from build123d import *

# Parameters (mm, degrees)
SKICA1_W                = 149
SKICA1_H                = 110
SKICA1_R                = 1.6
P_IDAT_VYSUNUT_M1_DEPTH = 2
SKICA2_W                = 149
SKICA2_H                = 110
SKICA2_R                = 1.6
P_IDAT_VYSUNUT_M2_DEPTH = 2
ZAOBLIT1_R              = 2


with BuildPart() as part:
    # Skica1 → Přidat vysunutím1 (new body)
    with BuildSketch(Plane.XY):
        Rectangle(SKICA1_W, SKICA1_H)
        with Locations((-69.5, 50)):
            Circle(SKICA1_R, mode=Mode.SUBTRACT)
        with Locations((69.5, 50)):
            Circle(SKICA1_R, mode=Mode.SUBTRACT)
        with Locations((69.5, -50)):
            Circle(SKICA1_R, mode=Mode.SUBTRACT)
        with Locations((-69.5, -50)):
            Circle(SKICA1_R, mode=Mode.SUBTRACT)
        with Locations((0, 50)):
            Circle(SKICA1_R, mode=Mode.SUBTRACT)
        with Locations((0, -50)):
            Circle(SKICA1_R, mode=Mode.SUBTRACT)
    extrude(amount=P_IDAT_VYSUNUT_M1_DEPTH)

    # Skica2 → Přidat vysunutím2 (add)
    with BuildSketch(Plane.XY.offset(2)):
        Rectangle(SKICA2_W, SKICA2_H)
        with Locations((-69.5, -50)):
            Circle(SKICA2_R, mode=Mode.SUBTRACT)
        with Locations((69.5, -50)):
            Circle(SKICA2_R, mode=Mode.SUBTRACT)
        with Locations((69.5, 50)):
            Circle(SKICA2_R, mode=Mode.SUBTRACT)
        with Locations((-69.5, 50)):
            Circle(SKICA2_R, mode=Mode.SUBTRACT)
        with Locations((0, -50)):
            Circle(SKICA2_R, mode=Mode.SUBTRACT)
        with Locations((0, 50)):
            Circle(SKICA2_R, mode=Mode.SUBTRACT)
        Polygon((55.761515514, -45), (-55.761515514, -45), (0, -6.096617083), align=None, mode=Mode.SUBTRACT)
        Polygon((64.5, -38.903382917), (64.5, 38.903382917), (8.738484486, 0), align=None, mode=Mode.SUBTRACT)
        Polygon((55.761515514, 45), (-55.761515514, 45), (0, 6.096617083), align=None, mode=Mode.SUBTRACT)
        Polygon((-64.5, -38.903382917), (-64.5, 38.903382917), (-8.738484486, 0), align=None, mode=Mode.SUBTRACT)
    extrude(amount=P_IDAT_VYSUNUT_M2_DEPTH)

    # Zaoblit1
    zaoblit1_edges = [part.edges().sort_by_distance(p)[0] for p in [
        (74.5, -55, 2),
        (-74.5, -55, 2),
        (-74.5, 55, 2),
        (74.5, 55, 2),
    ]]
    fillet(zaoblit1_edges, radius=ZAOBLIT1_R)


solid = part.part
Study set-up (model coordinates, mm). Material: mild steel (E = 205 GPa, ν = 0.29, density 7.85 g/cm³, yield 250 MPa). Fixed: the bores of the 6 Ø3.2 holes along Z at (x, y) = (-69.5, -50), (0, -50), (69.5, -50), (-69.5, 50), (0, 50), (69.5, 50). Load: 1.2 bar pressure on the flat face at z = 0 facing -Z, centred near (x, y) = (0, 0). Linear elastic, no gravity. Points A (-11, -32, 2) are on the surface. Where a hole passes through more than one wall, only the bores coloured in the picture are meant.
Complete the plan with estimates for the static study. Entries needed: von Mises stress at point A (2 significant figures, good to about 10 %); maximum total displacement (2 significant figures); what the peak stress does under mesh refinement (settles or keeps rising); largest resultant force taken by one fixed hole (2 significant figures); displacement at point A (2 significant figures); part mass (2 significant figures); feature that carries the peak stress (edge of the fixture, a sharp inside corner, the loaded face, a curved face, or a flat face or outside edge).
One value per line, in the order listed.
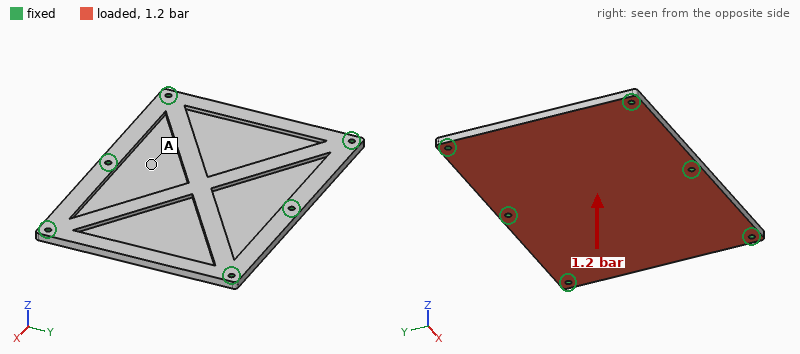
18 MPa
0.13 mm
keeps rising
540 N
0.056 mm
380 g
edge of the fixture
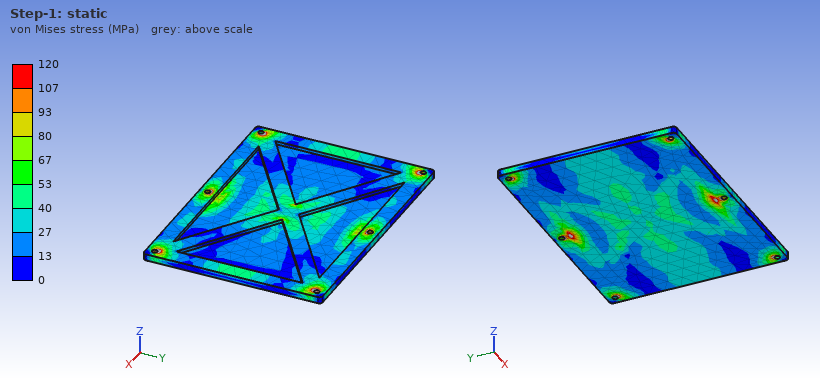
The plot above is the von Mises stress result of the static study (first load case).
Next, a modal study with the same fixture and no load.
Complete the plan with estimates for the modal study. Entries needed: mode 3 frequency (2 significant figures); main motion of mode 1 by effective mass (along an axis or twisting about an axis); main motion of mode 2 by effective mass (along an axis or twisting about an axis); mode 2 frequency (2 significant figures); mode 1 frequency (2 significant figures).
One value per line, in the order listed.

2400 Hz
along Z
twisting about Y
1700 Hz
1300 Hz
